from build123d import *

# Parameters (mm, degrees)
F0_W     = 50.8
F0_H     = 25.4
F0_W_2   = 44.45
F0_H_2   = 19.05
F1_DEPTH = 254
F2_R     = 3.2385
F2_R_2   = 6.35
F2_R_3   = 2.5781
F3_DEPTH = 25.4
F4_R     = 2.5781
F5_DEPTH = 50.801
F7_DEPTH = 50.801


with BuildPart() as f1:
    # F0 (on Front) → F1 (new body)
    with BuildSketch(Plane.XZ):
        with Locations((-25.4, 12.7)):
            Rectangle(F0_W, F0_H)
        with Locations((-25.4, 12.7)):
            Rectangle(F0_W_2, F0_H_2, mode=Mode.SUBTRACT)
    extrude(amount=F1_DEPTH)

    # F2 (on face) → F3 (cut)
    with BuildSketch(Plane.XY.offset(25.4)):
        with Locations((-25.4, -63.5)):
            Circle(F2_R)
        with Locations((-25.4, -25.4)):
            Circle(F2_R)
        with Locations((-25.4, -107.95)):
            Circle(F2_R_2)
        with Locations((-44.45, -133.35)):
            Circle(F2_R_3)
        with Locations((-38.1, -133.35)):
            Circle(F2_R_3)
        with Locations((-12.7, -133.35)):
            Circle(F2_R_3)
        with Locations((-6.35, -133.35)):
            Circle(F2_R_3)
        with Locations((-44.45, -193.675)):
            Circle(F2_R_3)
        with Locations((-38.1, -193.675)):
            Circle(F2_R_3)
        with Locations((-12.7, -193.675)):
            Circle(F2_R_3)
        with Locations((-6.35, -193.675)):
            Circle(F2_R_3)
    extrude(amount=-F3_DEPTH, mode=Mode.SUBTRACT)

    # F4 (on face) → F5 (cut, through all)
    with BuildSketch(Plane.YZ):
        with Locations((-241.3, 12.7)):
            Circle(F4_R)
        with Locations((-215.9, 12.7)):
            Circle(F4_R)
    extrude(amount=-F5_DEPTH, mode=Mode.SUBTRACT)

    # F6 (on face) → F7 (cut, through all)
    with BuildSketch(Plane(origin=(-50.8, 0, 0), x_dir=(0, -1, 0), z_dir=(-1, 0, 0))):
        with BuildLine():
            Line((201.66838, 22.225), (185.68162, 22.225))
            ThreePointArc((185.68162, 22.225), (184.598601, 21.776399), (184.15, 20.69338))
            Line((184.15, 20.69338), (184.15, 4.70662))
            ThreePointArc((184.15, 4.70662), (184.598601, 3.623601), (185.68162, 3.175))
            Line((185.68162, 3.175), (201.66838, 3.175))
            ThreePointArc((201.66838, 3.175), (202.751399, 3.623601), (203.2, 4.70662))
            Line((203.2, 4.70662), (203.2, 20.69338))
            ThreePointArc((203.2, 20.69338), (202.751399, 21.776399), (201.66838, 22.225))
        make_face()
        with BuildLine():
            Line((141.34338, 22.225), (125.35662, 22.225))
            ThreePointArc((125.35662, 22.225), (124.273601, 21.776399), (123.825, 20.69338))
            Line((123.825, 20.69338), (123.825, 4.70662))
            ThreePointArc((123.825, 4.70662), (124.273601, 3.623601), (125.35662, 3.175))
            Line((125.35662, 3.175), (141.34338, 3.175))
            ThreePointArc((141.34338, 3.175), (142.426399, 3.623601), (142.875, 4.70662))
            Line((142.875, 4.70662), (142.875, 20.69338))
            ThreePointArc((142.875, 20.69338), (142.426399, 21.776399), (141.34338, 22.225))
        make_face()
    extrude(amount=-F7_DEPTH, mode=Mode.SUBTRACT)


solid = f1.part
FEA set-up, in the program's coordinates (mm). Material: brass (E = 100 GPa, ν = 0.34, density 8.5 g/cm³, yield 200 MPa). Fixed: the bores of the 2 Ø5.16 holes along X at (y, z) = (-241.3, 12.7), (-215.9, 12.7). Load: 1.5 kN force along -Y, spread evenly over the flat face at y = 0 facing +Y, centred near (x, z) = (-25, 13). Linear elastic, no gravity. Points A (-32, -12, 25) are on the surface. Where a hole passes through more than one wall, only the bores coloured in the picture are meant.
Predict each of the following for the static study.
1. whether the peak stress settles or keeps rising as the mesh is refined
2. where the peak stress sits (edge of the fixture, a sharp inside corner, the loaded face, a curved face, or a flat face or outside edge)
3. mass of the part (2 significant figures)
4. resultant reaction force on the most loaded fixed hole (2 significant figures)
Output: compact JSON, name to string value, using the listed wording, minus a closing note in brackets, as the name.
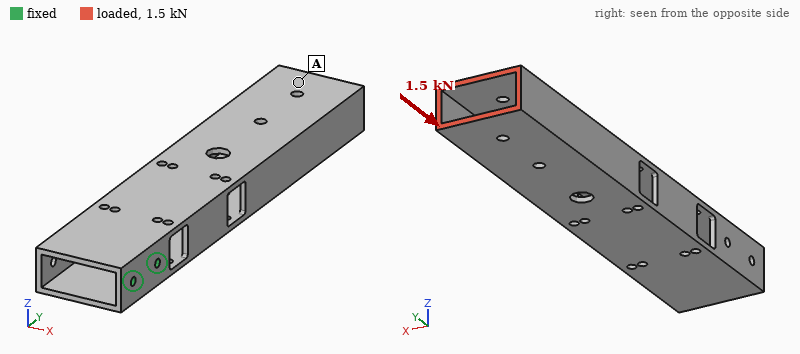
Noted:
{"whether the peak stress settles or keeps rising as the mesh is refined": "keeps rising", "where the peak stress sits": "edge of the fixture", "mass of the part": "900 g", "resultant reaction force on the most loaded fixed hole": "1.4 kN"}
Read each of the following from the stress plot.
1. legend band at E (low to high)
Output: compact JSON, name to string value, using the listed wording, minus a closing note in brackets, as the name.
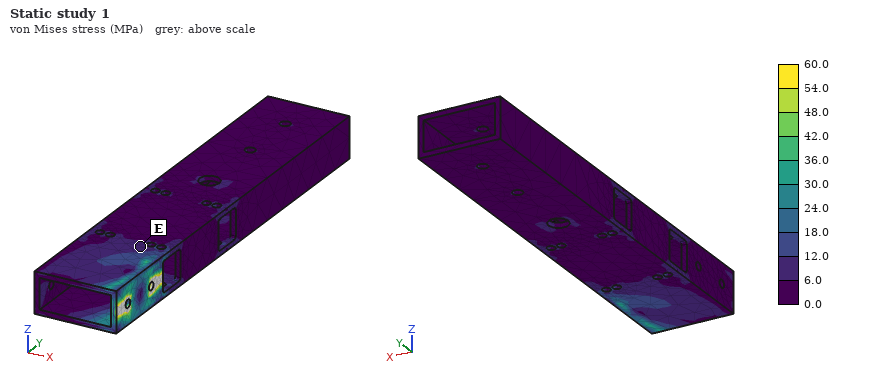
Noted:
{"legend band at E": "6.0 to 12.0 MPa"}
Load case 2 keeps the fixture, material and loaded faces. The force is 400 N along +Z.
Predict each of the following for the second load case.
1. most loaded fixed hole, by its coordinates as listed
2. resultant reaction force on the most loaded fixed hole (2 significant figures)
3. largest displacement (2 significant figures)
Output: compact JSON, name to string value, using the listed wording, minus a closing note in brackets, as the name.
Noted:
{"most loaded fixed hole, by its coordinates as listed": "(-215.9, 12.7)", "resultant reaction force on the most loaded fixed hole": "3.1 kN", "largest displacement": "1.1 mm"}
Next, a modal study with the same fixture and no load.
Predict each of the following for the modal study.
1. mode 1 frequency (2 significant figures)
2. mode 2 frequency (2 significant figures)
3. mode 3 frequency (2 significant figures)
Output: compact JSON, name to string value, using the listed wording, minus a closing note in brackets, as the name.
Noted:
{"mode 1 frequency": "180 Hz", "mode 2 frequency": "190 Hz", "mode 3 frequency": "420 Hz"}
